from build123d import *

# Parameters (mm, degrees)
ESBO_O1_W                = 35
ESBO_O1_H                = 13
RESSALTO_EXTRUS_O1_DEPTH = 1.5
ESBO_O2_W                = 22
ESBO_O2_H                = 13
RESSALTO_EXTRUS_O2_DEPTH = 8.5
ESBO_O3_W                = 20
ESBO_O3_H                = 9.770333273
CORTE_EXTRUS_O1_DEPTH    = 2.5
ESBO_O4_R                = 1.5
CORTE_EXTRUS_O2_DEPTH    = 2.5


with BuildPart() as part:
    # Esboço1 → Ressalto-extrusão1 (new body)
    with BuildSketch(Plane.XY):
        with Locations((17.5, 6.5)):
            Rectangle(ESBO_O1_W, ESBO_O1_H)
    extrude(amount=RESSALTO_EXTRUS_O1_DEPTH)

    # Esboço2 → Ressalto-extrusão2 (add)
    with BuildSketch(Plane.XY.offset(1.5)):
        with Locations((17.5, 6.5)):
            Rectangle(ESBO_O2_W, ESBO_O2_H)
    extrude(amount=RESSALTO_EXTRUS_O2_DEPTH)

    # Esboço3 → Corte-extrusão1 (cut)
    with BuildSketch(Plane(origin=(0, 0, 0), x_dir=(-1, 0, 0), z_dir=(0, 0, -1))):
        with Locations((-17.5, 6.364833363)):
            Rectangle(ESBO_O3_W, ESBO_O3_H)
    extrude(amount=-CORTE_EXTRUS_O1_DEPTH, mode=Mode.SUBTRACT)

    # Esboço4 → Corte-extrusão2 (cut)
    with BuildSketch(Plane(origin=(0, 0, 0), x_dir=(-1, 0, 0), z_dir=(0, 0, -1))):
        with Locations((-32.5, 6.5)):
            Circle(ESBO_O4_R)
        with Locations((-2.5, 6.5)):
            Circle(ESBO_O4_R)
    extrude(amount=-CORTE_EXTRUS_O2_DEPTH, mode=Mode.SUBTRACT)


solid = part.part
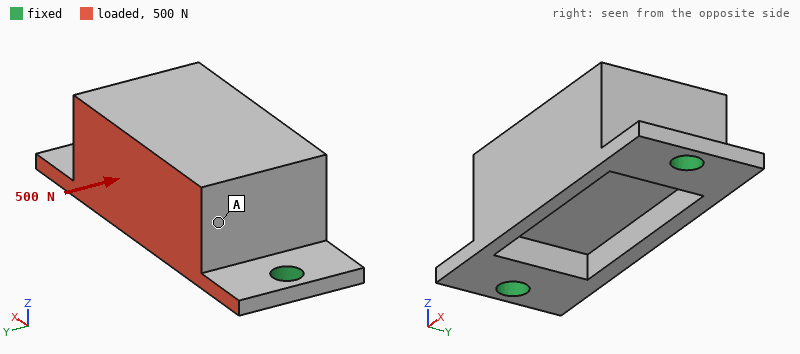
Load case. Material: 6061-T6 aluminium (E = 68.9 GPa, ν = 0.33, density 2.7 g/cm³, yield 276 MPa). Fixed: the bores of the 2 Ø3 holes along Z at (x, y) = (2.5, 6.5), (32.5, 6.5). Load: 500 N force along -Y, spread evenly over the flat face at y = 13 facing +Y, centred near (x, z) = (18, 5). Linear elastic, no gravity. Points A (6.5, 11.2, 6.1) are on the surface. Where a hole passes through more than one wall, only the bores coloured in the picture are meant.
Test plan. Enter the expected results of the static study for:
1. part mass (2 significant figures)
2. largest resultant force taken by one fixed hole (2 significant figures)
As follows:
7.0 g
250 N
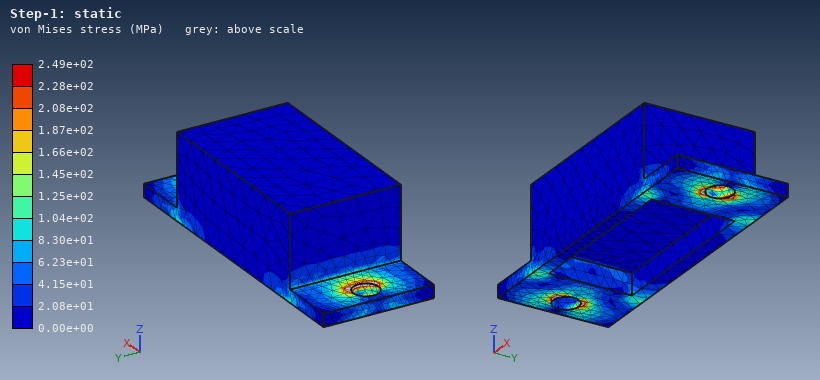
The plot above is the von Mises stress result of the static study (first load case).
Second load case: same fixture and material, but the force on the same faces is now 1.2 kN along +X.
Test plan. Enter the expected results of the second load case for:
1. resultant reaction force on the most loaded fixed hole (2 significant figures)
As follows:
670 N
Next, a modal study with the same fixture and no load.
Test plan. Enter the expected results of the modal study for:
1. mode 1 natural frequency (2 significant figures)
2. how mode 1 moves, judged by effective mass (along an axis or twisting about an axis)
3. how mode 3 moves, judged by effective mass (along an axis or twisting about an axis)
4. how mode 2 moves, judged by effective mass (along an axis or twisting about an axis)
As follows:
4700 Hz
along Y
along X
along Z
